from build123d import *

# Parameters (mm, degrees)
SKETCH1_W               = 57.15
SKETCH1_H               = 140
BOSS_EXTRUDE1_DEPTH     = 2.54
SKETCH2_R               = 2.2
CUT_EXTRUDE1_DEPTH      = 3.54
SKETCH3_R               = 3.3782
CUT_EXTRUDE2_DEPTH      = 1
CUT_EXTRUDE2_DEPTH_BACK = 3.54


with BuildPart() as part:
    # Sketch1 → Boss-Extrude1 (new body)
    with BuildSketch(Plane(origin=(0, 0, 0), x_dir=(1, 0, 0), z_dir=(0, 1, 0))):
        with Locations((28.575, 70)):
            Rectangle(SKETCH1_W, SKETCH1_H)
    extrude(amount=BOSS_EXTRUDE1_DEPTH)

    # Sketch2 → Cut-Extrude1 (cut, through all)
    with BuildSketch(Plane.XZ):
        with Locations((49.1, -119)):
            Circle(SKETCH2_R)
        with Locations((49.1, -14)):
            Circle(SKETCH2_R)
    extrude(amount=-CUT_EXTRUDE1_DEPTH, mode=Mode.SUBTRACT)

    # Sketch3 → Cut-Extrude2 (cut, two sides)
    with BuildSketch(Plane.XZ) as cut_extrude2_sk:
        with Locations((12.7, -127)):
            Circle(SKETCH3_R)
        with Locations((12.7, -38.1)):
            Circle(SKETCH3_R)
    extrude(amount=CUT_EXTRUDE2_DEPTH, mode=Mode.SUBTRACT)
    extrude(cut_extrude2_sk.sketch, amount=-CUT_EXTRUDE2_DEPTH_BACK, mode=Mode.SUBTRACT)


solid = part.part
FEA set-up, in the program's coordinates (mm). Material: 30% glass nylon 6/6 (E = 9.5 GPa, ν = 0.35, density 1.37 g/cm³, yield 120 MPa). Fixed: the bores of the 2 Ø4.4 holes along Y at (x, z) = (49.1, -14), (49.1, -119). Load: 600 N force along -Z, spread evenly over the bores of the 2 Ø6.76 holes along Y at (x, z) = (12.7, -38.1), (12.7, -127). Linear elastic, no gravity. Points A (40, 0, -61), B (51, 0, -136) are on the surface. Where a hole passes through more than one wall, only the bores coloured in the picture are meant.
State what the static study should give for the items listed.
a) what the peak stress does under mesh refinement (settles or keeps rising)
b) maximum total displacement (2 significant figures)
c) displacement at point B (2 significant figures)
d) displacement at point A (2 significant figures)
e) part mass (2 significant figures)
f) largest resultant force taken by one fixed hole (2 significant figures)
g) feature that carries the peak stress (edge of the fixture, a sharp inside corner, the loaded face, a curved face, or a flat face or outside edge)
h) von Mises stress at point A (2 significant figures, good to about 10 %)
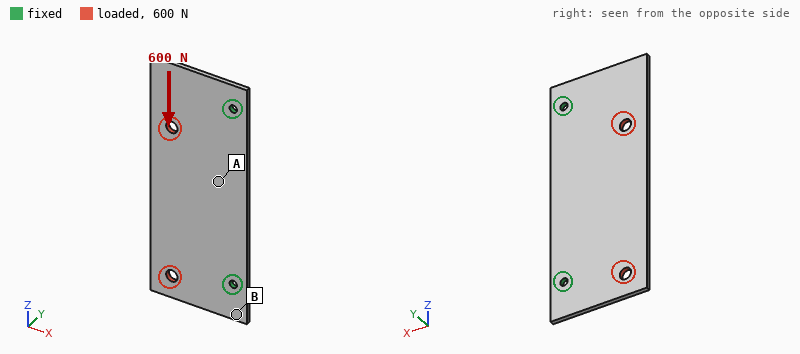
keeps rising
61 µm
23 µm
19 µm
27 g
360 N
edge of the fixture
2.9 MPa
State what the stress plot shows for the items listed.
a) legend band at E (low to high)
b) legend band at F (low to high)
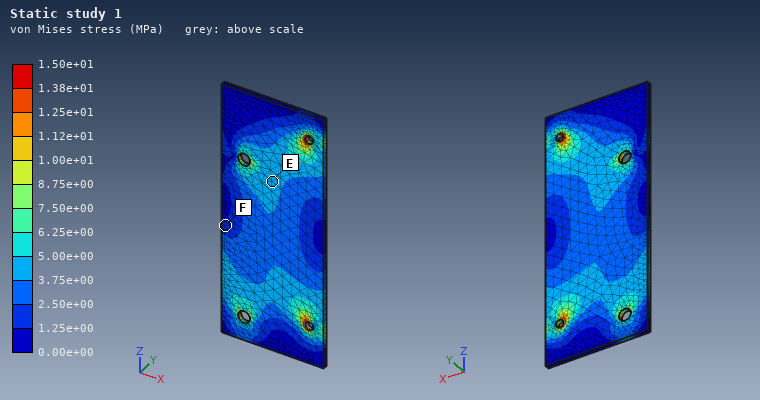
3.75e+00 to 5.00e+00 MPa
1.25e+00 to 2.50e+00 MPa
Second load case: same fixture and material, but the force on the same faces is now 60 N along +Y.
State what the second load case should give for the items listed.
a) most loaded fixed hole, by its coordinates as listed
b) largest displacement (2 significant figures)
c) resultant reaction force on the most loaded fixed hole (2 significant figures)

(49.1, -119)
1.6 mm
37 N
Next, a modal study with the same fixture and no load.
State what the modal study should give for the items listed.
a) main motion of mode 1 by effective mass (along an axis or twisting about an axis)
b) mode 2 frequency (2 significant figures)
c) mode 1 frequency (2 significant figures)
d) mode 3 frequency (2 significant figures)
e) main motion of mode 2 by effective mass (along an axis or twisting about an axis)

along Y
540 Hz
300 Hz
620 Hz
twisting about X
